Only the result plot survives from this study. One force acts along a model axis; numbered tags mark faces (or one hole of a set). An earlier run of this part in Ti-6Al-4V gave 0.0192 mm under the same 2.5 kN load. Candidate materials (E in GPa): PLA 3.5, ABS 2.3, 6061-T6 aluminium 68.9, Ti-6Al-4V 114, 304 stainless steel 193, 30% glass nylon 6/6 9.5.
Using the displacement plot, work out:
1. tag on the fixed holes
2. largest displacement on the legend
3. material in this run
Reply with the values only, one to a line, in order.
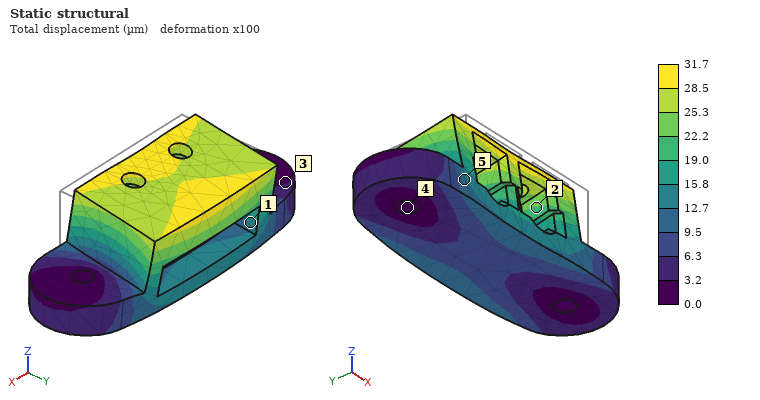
4
31.7 µm
6061-T6 aluminium
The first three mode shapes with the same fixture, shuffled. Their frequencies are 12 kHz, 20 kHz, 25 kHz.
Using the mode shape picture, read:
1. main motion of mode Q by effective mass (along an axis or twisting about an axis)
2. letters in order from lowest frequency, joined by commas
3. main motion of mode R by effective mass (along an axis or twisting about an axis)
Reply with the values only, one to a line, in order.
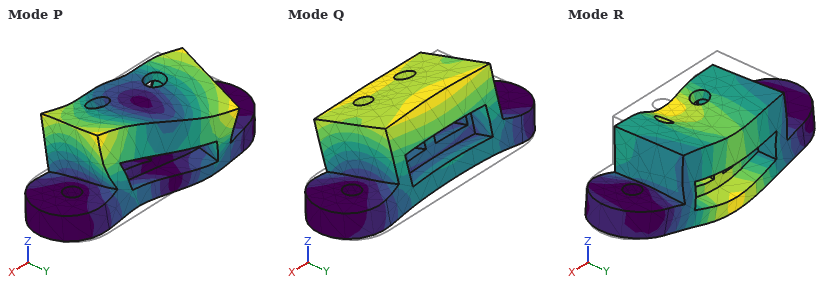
along Y
Q, R, P
along Z
